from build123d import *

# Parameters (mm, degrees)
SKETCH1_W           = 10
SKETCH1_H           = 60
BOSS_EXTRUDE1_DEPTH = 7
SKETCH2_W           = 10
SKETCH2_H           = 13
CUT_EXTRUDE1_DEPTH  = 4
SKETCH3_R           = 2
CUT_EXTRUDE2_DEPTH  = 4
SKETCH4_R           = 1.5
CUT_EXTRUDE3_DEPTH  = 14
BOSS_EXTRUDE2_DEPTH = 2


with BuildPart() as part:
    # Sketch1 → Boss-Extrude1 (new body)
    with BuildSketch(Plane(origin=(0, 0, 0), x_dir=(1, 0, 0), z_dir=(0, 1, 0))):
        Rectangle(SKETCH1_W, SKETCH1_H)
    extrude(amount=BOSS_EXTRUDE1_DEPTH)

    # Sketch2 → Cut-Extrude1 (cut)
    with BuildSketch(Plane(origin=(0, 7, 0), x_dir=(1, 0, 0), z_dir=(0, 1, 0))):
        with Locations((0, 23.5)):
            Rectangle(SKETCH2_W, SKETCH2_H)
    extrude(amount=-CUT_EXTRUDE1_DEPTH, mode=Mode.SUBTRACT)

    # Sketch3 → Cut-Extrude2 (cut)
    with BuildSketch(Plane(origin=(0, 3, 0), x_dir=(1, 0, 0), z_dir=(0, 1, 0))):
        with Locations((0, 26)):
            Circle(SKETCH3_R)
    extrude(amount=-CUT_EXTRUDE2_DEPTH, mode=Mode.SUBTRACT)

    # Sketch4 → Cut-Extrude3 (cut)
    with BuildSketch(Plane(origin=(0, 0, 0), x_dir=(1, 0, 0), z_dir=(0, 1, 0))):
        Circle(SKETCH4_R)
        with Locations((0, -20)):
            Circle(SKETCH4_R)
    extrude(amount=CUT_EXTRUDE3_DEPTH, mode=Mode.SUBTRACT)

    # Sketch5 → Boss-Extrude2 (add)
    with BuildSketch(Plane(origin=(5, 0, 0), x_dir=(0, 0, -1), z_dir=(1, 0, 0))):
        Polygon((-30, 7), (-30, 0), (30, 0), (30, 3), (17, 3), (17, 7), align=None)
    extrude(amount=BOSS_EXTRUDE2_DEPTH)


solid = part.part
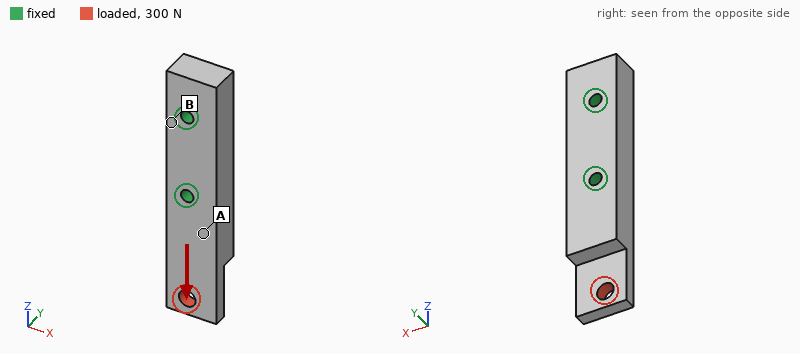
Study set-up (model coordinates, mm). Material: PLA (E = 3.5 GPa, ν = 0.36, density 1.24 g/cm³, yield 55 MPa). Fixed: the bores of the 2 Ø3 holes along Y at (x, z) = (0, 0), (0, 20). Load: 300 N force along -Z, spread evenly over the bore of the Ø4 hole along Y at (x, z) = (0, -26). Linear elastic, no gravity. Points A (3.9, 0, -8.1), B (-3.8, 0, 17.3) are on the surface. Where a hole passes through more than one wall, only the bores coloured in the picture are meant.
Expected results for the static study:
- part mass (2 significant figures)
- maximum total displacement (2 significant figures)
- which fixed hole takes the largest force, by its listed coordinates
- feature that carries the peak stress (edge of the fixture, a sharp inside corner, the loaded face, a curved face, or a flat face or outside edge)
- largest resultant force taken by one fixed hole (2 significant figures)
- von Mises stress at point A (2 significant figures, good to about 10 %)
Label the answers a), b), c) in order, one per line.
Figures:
a) 5.3 g
b) 0.22 mm
c) (0, 0)
d) the loaded face
e) 270 N
f) 8.6 MPa
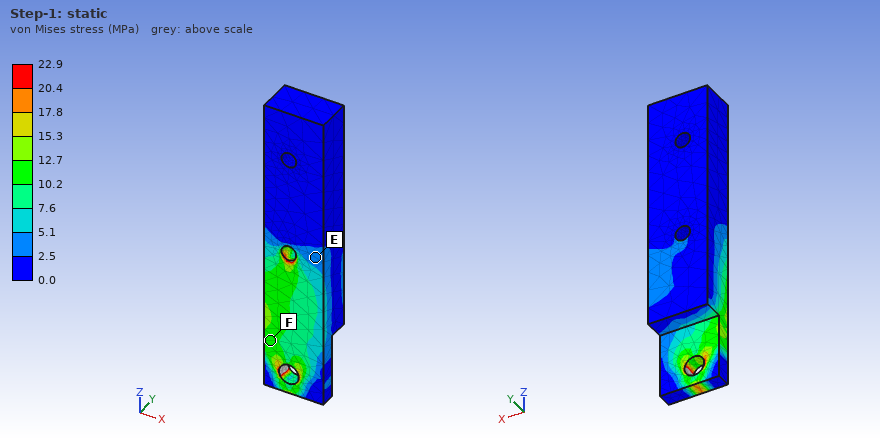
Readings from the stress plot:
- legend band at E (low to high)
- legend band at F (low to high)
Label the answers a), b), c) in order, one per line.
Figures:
a) 2.5 to 5.1 MPa
b) 10.2 to 12.7 MPa
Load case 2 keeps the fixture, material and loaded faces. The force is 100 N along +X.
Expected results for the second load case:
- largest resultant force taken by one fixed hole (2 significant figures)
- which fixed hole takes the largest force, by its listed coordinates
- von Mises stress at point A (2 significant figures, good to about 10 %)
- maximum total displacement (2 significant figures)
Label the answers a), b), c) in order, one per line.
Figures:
a) 190 N
b) (0, 0)
c) 6.8 MPa
d) 0.42 mm
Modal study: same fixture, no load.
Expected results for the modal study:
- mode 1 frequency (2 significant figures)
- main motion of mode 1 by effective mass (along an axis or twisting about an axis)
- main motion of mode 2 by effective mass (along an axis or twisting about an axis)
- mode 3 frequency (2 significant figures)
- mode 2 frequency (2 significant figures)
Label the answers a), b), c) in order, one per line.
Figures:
a) 2600 Hz
b) along Y
c) along X
d) 7000 Hz
e) 3700 Hz
